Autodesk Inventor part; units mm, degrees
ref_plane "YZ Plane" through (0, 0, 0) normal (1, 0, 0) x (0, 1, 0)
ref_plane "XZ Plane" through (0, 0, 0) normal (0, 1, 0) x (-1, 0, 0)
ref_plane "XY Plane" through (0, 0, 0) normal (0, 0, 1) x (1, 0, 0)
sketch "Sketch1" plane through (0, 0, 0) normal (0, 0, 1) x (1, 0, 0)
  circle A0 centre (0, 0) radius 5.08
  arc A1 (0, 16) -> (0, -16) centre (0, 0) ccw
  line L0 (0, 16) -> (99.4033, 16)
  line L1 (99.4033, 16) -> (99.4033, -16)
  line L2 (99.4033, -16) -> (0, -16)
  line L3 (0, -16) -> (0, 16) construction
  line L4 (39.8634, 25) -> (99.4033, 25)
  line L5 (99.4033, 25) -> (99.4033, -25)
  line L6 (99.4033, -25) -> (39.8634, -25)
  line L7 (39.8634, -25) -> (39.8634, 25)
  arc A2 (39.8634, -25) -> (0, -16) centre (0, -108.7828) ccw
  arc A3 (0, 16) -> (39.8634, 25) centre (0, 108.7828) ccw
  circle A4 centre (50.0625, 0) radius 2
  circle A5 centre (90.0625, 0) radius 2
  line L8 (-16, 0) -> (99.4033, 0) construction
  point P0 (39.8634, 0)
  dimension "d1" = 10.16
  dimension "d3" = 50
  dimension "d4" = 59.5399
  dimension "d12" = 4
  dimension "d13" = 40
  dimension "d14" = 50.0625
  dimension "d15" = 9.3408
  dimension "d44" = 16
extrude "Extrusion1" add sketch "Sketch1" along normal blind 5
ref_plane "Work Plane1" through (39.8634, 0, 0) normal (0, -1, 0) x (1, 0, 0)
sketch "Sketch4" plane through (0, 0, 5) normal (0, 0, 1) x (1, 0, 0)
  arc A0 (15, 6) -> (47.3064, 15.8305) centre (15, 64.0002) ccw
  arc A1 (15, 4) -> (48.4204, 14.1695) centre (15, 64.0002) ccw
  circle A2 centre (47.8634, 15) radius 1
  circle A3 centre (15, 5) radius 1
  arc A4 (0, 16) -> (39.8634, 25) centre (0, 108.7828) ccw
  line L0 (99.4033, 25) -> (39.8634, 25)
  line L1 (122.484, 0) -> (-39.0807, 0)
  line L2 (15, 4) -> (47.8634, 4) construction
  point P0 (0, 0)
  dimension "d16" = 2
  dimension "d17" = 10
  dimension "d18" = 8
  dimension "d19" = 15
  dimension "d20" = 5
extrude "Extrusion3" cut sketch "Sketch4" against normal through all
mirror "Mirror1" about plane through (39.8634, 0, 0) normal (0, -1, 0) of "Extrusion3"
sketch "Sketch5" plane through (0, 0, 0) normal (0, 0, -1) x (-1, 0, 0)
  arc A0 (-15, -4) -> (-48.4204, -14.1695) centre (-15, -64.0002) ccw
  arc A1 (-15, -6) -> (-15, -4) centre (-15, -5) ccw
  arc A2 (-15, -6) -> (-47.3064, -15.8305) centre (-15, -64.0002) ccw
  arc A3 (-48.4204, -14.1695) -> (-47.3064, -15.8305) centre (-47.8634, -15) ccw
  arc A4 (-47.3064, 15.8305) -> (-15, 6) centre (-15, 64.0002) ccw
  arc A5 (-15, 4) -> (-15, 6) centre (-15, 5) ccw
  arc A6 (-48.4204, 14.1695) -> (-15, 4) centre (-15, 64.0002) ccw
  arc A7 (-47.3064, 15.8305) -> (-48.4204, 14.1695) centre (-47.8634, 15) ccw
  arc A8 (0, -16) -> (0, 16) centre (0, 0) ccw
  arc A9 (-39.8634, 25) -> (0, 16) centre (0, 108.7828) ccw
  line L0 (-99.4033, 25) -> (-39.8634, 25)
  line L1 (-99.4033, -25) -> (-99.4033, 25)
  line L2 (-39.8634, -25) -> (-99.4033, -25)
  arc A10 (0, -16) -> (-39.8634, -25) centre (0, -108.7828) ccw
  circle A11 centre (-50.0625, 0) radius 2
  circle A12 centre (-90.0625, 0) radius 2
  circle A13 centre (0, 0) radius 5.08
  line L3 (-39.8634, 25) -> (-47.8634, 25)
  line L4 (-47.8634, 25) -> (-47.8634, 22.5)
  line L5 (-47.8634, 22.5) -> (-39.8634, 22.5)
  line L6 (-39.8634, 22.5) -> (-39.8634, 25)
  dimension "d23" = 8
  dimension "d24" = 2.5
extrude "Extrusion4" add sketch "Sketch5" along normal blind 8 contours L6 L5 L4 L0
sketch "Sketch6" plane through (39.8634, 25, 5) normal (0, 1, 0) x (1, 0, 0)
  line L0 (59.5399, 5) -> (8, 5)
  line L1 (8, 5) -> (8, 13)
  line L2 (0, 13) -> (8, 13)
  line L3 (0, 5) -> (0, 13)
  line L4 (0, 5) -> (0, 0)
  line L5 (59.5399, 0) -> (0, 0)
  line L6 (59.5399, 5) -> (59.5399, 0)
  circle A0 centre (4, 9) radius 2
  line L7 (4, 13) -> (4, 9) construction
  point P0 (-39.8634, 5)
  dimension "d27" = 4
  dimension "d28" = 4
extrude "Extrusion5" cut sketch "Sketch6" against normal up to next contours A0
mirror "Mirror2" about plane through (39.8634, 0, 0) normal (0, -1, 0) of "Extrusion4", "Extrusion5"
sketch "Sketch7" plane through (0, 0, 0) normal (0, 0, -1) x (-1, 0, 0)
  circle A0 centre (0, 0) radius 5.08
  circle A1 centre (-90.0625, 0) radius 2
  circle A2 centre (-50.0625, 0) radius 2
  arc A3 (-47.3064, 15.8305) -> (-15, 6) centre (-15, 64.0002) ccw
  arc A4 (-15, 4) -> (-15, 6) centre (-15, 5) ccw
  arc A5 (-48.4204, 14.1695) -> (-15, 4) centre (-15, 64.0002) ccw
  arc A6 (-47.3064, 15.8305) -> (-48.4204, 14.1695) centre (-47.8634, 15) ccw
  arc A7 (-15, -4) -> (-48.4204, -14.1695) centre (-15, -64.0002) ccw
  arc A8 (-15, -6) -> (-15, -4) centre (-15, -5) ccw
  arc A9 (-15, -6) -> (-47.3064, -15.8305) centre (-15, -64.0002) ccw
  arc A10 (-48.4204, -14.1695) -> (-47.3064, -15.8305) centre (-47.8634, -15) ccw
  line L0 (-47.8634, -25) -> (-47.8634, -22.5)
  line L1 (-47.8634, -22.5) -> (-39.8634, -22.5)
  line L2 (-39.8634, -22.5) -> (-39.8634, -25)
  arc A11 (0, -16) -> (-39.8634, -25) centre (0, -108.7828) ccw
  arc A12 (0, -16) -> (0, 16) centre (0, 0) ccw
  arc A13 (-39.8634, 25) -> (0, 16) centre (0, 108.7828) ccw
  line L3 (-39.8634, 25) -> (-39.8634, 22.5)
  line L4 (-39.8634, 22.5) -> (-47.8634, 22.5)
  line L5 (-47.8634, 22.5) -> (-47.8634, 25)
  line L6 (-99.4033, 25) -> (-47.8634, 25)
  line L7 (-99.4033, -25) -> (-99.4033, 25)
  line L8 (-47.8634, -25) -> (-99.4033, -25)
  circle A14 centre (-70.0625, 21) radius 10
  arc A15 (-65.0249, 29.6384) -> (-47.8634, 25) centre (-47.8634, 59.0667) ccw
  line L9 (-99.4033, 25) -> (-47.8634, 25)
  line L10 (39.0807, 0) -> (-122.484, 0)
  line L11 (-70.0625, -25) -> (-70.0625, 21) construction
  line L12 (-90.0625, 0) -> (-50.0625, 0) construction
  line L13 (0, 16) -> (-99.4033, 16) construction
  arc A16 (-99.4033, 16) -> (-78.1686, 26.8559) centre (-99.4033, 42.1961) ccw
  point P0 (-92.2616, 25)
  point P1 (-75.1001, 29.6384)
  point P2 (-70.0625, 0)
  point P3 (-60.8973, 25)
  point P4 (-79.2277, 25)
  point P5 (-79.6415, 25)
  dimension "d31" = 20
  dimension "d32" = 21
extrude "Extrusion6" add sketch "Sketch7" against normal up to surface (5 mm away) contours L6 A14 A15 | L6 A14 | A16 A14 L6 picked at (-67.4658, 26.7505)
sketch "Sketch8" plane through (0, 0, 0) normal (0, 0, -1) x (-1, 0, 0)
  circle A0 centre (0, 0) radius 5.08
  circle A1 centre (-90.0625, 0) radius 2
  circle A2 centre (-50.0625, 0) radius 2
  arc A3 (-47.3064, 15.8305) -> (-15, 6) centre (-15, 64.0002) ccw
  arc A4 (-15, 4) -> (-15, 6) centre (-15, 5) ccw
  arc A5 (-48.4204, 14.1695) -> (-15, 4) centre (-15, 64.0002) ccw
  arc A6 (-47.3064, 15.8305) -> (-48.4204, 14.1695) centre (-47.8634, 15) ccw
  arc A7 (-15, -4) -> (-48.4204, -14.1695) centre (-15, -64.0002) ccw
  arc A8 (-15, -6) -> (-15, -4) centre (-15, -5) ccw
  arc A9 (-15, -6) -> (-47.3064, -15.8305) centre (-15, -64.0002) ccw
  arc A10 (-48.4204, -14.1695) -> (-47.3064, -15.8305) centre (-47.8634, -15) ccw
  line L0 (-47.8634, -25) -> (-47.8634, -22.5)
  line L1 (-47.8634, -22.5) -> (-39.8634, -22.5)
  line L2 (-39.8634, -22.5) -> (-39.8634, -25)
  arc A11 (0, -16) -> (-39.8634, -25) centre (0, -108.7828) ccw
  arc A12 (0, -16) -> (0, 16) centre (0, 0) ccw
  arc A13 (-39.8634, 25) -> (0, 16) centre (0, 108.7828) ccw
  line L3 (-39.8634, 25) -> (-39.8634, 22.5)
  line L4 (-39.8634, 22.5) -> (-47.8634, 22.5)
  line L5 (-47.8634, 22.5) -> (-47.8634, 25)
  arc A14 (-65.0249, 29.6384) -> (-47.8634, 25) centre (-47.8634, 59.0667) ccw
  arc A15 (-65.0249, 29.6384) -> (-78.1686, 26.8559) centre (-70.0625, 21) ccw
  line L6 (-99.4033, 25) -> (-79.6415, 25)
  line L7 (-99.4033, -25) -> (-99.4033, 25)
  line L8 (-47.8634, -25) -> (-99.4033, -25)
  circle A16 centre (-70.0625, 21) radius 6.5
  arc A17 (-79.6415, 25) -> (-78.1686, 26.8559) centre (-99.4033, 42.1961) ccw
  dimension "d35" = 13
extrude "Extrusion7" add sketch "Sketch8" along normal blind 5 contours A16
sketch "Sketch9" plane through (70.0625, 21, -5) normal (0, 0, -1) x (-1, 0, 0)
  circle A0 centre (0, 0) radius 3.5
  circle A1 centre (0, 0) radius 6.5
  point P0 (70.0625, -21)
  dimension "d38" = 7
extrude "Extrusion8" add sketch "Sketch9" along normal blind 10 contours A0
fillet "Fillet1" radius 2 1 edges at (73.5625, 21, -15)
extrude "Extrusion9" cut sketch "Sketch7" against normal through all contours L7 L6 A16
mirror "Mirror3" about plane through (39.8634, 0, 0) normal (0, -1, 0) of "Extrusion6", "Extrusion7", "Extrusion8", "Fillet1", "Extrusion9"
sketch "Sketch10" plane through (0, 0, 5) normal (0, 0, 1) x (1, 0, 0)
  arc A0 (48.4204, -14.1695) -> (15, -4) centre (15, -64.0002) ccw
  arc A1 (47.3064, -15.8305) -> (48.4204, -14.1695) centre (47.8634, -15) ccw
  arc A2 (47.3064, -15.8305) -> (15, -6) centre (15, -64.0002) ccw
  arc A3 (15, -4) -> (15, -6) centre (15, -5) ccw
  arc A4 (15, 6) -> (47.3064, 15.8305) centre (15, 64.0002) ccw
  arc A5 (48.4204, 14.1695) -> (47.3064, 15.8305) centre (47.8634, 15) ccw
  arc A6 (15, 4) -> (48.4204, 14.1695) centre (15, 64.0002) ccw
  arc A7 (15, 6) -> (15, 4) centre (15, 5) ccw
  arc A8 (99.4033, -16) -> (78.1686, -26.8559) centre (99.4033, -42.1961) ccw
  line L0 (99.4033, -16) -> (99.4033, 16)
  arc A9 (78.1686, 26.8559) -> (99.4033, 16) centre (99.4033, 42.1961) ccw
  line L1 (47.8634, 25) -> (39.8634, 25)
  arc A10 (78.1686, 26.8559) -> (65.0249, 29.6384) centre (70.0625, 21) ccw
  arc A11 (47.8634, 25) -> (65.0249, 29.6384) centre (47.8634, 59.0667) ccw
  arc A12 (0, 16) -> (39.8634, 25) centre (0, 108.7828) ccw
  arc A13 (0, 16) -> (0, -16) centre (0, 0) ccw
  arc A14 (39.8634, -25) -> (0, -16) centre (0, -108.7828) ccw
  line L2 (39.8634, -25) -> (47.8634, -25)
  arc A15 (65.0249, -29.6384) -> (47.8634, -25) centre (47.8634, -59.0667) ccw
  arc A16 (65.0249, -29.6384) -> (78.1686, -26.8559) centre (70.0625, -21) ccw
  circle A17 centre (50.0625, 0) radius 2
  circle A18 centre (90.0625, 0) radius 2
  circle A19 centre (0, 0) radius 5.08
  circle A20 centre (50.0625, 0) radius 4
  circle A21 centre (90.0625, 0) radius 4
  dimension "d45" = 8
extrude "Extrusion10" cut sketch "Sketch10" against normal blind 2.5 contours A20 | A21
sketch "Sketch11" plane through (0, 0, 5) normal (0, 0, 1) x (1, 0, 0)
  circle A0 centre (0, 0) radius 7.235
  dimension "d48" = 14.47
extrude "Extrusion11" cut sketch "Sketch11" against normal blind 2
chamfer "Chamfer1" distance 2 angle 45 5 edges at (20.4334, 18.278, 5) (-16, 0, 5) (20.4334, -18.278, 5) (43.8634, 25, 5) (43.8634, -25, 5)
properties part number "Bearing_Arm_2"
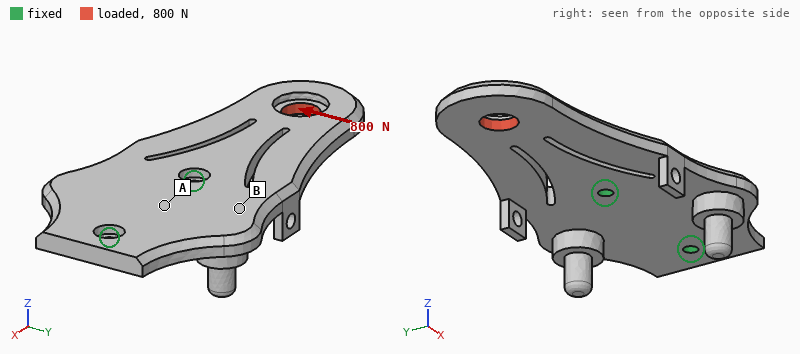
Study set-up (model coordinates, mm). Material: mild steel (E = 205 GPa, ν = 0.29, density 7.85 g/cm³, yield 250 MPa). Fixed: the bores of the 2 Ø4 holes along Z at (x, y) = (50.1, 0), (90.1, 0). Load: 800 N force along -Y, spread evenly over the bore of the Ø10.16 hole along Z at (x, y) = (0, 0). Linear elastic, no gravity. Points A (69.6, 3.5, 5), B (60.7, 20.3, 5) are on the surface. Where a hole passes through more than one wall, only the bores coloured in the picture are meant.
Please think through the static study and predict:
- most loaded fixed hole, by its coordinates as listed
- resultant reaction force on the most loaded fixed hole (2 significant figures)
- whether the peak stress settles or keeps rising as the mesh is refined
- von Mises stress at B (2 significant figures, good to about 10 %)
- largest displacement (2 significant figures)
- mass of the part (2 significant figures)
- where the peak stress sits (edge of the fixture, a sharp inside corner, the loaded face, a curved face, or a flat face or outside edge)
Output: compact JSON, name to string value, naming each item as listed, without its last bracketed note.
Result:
{"most loaded fixed hole, by its coordinates as listed": "(50.1, 0)", "resultant reaction force on the most loaded fixed hole": "1.7 kN", "whether the peak stress settles or keeps rising as the mesh is refined": "keeps rising", "von Mises stress at B": "13 MPa", "largest displacement": "25 µm", "mass of the part": "190 g", "where the peak stress sits": "edge of the fixture"}
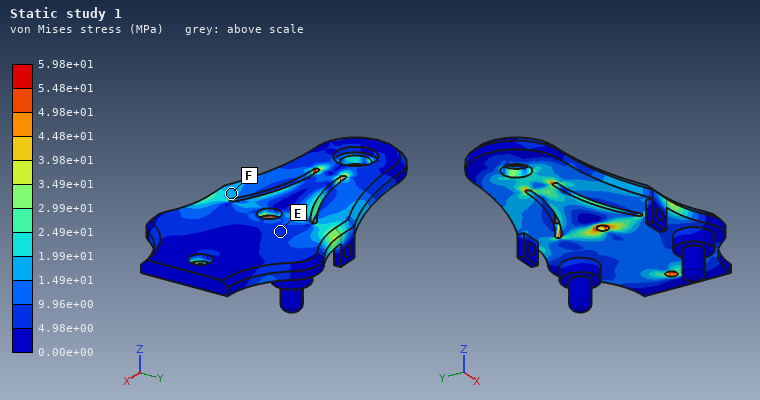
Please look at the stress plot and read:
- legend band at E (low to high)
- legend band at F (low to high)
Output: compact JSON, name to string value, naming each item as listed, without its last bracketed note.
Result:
{"legend band at E": "4.98e+00 to 9.96e+00 MPa", "legend band at F": "1.49e+01 to 1.99e+01 MPa"}
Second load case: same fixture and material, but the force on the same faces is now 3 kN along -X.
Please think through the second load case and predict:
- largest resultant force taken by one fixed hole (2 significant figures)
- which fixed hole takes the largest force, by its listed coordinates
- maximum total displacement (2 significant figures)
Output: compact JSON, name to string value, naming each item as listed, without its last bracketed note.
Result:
{"largest resultant force taken by one fixed hole": "2.1 kN", "which fixed hole takes the largest force, by its listed coordinates": "(50.1, 0)", "maximum total displacement": "82 µm"}
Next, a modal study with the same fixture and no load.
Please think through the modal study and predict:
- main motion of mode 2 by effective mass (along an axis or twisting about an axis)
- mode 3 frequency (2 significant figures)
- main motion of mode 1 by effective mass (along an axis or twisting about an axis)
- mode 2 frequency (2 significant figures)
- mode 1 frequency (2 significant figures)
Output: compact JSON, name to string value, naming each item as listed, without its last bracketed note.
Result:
{"main motion of mode 2 by effective mass": "twisting about X", "mode 3 frequency": "3900 Hz", "main motion of mode 1 by effective mass": "along Z", "mode 2 frequency": "2000 Hz", "mode 1 frequency": "1000 Hz"}
